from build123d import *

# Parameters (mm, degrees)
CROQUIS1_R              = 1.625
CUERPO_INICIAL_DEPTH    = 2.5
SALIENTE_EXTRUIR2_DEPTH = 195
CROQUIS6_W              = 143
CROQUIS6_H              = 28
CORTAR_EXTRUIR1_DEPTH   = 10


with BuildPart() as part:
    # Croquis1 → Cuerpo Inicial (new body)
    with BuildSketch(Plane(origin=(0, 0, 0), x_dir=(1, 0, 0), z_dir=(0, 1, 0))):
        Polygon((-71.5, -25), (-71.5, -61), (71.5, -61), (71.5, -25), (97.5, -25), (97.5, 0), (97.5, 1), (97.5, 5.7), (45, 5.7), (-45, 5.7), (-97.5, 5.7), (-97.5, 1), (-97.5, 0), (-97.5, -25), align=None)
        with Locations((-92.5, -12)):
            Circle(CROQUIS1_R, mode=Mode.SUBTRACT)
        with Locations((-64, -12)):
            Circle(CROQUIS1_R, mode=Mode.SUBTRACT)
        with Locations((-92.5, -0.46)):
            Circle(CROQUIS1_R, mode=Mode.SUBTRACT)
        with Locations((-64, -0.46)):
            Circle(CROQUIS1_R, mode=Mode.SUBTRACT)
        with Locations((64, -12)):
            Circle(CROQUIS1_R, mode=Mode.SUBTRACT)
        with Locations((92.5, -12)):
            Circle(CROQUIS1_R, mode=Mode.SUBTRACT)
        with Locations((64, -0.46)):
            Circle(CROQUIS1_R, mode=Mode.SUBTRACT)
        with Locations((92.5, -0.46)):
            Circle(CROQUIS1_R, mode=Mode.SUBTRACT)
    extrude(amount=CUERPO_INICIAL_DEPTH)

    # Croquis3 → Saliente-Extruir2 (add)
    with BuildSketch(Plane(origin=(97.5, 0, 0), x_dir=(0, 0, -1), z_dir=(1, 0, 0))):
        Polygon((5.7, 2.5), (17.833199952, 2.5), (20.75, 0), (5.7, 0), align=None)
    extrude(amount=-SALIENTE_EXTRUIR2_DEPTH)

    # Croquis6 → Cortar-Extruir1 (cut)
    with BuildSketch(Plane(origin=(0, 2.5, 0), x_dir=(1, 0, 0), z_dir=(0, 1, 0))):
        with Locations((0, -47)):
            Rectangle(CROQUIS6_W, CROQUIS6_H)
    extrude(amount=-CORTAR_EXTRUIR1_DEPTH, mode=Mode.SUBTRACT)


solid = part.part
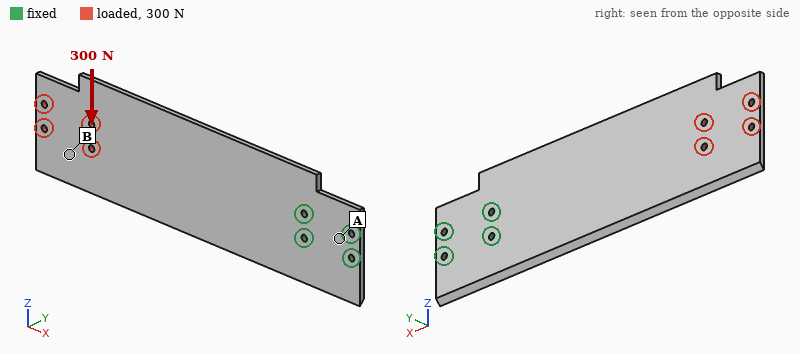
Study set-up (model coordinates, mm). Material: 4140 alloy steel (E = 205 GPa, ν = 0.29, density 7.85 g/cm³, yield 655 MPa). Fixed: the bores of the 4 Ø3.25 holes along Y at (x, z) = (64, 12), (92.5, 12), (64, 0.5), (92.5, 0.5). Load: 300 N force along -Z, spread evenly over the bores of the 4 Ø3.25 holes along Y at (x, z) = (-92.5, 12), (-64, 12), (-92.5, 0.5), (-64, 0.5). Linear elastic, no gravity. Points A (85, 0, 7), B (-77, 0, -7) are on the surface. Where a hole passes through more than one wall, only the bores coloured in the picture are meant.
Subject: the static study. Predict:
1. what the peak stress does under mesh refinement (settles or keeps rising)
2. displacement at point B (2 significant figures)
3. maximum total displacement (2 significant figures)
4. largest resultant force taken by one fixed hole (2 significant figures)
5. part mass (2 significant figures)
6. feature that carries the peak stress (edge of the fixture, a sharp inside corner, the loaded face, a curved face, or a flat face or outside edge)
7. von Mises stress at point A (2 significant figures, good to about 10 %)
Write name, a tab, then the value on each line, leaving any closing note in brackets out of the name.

what the peak stress does under mesh refinement	keeps rising
displacement at point B	0.087 mm
maximum total displacement	0.10 mm
largest resultant force taken by one fixed hole	1.2 kN
part mass	190 g
feature that carries the peak stress	edge of the fixture
von Mises stress at point A	12 MPa
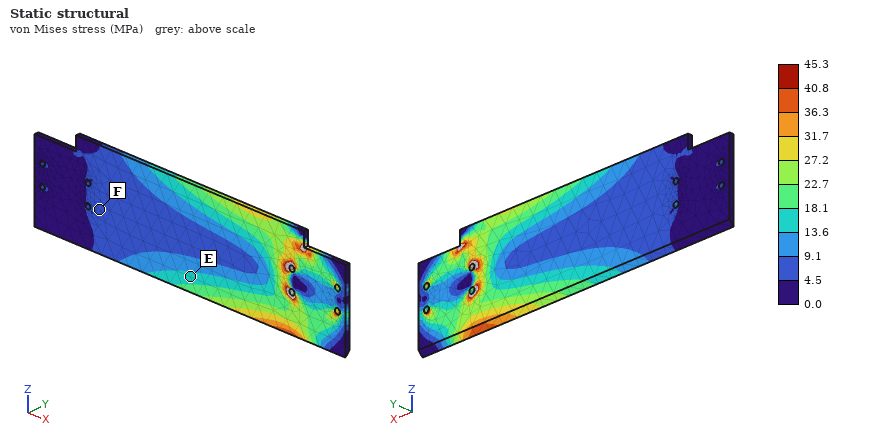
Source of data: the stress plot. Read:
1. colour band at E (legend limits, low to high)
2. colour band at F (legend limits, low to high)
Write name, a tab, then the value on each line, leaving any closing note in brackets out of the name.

colour band at E	13.6 to 18.1 MPa
colour band at F	4.5 to 9.1 MPa
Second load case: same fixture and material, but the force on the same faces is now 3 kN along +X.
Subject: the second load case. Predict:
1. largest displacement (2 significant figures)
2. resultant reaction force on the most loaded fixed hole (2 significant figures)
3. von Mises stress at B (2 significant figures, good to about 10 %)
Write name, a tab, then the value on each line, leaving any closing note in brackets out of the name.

largest displacement	35 µm
resultant reaction force on the most loaded fixed hole	1.3 kN
von Mises stress at B	17 MPa
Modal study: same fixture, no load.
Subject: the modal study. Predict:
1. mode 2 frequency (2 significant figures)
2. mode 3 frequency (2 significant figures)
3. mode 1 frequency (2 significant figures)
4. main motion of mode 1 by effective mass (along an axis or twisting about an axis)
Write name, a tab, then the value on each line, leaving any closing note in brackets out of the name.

mode 2 frequency	490 Hz
mode 3 frequency	530 Hz
mode 1 frequency	82 Hz
main motion of mode 1 by effective mass	along Y
